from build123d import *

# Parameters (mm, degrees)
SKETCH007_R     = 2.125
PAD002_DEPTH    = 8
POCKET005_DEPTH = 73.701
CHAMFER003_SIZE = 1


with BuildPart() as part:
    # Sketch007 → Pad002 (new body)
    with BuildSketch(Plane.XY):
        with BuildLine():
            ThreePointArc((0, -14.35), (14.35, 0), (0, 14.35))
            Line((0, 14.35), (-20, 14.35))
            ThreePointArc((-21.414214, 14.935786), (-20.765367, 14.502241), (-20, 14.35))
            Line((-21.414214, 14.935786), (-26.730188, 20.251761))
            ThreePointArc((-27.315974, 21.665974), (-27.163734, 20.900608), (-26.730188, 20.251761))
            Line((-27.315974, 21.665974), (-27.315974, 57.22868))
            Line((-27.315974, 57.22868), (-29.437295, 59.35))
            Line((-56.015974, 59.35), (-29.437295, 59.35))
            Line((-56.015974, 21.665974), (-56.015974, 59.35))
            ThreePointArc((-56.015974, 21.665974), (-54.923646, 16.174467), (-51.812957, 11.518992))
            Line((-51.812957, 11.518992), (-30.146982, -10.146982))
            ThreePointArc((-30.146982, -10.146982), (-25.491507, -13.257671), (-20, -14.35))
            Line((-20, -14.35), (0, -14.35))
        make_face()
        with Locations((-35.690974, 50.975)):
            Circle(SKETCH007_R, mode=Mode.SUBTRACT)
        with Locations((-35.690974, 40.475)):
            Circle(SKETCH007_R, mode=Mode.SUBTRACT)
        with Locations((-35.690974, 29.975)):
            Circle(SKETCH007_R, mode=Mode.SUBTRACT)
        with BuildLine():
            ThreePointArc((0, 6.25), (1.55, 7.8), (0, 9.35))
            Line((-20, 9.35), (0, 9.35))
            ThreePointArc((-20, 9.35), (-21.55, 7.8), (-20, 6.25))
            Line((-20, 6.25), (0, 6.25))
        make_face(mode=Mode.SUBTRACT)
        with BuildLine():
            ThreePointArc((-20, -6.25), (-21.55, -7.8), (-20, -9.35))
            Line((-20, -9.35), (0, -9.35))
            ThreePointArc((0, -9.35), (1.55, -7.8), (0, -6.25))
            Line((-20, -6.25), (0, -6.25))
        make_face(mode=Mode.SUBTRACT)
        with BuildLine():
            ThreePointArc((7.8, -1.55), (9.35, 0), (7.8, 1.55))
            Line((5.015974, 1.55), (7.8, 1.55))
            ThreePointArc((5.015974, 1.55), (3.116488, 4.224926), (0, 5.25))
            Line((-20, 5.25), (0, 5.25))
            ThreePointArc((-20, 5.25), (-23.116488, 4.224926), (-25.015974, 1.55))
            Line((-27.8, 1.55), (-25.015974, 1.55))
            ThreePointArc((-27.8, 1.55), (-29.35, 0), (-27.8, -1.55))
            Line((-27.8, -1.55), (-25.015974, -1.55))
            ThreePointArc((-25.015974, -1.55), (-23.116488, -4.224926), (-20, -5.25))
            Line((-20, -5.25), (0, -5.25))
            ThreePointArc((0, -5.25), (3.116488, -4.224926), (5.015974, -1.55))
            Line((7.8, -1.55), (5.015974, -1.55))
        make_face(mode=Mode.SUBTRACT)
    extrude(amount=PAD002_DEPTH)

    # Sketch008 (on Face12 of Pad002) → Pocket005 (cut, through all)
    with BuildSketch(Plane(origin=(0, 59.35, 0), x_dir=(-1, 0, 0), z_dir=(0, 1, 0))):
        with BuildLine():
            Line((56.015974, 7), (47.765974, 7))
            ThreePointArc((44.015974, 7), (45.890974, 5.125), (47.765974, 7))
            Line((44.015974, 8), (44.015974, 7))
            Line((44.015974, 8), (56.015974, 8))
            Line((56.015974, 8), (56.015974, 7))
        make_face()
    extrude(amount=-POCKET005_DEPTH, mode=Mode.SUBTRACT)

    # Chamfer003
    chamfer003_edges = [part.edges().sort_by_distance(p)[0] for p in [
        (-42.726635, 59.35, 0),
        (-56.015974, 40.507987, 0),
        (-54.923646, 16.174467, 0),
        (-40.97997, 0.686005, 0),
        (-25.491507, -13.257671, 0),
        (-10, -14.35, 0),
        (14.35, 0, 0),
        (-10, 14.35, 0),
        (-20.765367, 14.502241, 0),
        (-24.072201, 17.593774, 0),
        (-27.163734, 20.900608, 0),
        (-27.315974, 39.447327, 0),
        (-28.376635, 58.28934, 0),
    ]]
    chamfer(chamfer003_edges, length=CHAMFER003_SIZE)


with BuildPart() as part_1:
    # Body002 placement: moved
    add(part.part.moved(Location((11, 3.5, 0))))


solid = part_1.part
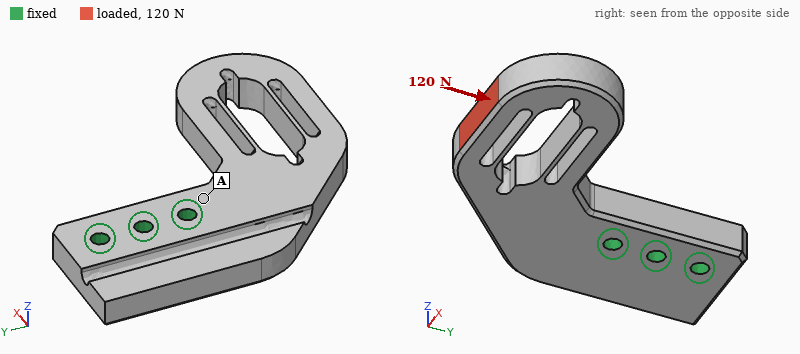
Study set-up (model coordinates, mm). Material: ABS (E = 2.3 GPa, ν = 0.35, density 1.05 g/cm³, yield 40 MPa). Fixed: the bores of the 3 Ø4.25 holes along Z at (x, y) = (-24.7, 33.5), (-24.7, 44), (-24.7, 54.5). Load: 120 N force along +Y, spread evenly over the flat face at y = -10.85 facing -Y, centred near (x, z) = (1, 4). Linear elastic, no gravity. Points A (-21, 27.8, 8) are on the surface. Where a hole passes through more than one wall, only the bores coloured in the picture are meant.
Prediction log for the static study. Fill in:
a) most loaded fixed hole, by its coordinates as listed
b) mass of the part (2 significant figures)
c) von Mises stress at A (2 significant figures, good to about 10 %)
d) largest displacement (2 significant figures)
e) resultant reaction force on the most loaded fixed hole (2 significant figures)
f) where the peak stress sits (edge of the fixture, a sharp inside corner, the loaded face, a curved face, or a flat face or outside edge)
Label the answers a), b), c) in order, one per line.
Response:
a) (-24.7, 33.5)
b) 18 g
c) 2.9 MPa
d) 0.89 mm
e) 200 N
f) a curved face
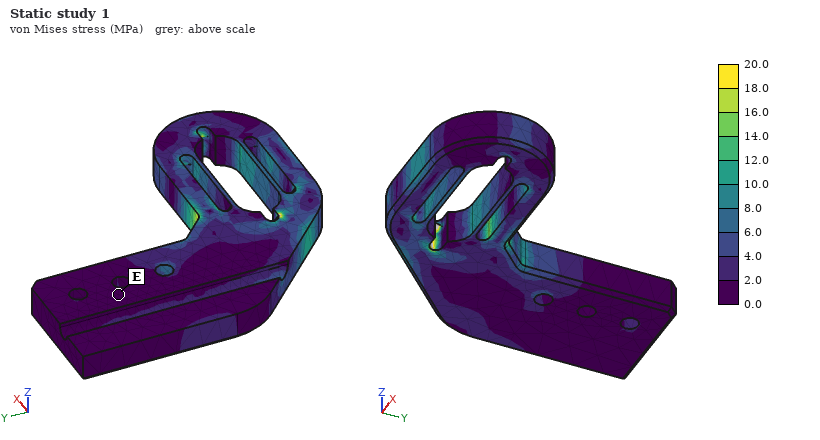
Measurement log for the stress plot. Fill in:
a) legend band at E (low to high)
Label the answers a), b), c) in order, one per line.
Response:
a) 0.0 to 2.0 MPa
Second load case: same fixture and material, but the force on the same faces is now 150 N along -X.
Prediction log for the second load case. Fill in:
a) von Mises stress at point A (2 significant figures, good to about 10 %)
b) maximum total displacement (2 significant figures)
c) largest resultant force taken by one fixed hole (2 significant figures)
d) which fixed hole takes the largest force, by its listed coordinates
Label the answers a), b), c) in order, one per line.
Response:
a) 2.9 MPa
b) 0.91 mm
c) 430 N
d) (-24.7, 33.5)
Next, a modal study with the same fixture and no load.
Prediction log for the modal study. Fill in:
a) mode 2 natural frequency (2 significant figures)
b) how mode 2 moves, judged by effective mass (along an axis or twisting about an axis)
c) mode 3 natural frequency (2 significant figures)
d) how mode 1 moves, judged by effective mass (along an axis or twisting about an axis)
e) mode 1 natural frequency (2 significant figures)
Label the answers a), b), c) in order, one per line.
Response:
a) 840 Hz
b) along Y
c) 1200 Hz
d) along Z
e) 470 Hz
